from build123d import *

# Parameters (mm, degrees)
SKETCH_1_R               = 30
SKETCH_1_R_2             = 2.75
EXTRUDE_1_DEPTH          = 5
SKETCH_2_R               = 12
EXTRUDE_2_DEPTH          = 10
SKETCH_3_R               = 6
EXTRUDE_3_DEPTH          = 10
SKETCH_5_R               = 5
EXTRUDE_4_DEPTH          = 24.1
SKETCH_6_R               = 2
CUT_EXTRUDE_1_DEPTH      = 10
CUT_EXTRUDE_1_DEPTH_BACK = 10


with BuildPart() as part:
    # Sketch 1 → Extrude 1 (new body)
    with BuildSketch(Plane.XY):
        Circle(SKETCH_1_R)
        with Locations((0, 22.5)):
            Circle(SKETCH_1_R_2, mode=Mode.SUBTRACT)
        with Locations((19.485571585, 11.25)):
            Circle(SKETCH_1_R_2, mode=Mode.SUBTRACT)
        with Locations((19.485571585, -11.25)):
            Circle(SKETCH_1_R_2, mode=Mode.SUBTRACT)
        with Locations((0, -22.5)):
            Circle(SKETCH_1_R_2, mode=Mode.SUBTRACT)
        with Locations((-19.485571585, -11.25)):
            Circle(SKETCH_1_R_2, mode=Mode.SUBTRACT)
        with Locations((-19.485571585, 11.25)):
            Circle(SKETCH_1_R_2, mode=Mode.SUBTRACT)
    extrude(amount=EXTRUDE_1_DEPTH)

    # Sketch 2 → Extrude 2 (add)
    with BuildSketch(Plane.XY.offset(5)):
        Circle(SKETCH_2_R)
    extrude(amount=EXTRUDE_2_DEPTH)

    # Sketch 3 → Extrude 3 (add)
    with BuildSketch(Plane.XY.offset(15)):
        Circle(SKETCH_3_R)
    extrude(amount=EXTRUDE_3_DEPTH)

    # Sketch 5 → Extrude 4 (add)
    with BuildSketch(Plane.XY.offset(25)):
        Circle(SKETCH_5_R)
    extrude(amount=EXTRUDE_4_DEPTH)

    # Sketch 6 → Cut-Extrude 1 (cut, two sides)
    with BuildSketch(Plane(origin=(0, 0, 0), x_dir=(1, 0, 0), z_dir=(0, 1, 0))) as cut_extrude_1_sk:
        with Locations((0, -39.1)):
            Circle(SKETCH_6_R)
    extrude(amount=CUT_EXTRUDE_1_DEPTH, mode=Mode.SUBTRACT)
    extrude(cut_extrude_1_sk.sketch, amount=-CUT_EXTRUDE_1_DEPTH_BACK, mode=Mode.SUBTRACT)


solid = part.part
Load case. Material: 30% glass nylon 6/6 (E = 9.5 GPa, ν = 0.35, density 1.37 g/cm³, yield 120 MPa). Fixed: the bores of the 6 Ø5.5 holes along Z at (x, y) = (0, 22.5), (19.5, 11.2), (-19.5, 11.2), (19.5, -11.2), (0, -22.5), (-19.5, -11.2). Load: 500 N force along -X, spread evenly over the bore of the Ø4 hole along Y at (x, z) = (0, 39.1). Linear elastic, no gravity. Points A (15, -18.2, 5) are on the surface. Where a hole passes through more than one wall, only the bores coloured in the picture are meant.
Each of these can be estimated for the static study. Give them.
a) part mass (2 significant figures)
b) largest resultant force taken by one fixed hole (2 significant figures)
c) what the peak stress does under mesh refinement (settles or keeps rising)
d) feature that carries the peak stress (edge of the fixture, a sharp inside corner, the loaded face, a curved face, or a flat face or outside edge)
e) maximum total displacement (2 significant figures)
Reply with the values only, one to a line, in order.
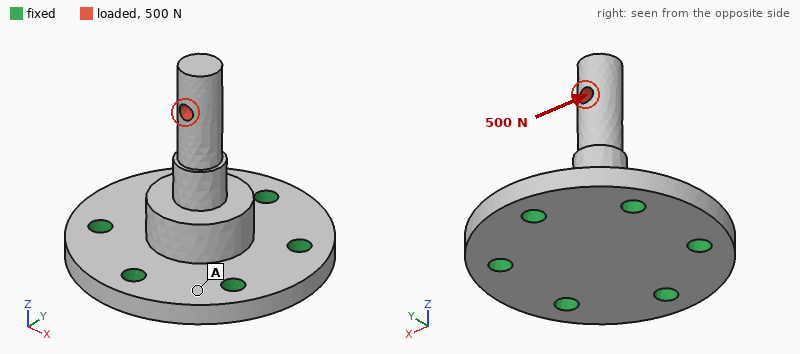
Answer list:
29 g
330 N
keeps rising
a sharp inside corner
0.81 mm
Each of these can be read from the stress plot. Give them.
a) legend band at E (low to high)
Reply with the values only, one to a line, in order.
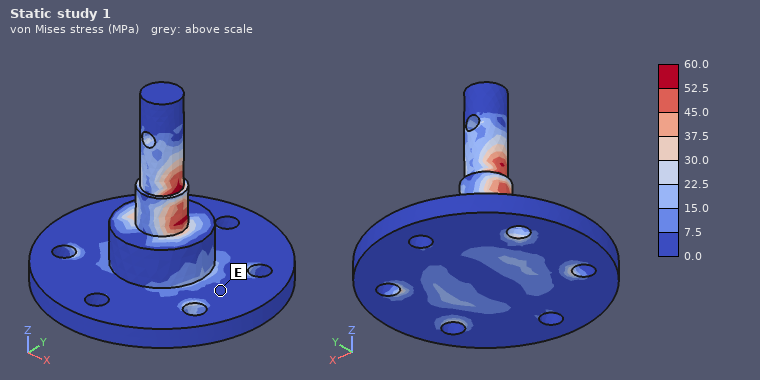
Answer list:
0.0 to 7.5 MPa
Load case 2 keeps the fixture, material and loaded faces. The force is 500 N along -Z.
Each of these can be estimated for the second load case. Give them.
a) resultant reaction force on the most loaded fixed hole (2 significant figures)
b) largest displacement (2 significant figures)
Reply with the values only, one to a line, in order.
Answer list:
92 N
31 µm
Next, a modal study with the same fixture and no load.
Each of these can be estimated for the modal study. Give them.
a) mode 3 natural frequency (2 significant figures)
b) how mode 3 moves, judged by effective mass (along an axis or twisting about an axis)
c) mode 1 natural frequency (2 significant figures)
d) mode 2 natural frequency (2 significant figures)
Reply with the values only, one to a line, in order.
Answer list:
8500 Hz
along Z
3100 Hz
3200 Hz
